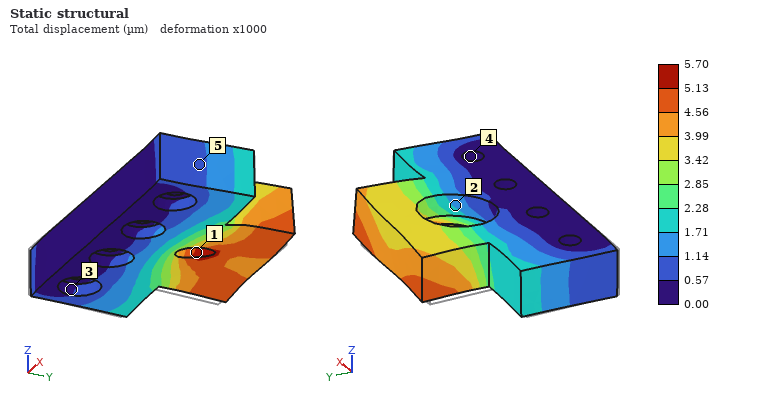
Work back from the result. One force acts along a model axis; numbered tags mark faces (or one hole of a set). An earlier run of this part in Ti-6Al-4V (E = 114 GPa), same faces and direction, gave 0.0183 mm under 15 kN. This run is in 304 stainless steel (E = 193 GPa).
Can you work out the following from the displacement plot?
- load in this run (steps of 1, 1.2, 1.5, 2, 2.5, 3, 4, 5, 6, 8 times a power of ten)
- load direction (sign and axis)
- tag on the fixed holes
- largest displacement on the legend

8 kN
+X
4
5.70 µm
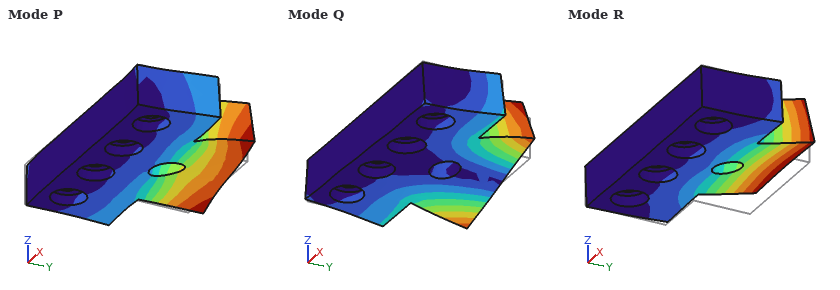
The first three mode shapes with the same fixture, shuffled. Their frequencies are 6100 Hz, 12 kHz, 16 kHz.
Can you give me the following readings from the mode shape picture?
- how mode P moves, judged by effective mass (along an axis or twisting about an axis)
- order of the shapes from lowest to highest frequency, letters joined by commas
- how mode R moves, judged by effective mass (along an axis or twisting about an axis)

along X
R, Q, P
along Z
